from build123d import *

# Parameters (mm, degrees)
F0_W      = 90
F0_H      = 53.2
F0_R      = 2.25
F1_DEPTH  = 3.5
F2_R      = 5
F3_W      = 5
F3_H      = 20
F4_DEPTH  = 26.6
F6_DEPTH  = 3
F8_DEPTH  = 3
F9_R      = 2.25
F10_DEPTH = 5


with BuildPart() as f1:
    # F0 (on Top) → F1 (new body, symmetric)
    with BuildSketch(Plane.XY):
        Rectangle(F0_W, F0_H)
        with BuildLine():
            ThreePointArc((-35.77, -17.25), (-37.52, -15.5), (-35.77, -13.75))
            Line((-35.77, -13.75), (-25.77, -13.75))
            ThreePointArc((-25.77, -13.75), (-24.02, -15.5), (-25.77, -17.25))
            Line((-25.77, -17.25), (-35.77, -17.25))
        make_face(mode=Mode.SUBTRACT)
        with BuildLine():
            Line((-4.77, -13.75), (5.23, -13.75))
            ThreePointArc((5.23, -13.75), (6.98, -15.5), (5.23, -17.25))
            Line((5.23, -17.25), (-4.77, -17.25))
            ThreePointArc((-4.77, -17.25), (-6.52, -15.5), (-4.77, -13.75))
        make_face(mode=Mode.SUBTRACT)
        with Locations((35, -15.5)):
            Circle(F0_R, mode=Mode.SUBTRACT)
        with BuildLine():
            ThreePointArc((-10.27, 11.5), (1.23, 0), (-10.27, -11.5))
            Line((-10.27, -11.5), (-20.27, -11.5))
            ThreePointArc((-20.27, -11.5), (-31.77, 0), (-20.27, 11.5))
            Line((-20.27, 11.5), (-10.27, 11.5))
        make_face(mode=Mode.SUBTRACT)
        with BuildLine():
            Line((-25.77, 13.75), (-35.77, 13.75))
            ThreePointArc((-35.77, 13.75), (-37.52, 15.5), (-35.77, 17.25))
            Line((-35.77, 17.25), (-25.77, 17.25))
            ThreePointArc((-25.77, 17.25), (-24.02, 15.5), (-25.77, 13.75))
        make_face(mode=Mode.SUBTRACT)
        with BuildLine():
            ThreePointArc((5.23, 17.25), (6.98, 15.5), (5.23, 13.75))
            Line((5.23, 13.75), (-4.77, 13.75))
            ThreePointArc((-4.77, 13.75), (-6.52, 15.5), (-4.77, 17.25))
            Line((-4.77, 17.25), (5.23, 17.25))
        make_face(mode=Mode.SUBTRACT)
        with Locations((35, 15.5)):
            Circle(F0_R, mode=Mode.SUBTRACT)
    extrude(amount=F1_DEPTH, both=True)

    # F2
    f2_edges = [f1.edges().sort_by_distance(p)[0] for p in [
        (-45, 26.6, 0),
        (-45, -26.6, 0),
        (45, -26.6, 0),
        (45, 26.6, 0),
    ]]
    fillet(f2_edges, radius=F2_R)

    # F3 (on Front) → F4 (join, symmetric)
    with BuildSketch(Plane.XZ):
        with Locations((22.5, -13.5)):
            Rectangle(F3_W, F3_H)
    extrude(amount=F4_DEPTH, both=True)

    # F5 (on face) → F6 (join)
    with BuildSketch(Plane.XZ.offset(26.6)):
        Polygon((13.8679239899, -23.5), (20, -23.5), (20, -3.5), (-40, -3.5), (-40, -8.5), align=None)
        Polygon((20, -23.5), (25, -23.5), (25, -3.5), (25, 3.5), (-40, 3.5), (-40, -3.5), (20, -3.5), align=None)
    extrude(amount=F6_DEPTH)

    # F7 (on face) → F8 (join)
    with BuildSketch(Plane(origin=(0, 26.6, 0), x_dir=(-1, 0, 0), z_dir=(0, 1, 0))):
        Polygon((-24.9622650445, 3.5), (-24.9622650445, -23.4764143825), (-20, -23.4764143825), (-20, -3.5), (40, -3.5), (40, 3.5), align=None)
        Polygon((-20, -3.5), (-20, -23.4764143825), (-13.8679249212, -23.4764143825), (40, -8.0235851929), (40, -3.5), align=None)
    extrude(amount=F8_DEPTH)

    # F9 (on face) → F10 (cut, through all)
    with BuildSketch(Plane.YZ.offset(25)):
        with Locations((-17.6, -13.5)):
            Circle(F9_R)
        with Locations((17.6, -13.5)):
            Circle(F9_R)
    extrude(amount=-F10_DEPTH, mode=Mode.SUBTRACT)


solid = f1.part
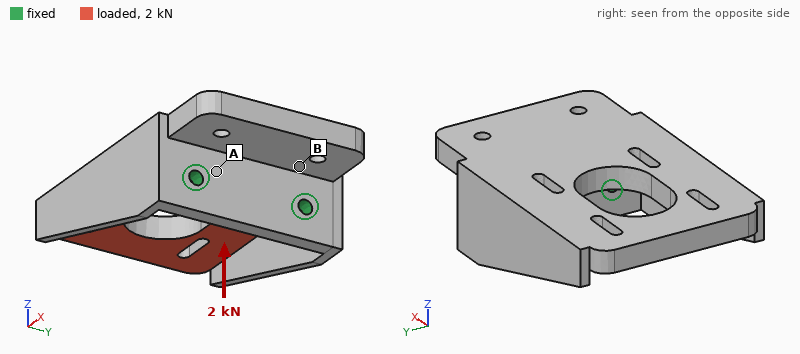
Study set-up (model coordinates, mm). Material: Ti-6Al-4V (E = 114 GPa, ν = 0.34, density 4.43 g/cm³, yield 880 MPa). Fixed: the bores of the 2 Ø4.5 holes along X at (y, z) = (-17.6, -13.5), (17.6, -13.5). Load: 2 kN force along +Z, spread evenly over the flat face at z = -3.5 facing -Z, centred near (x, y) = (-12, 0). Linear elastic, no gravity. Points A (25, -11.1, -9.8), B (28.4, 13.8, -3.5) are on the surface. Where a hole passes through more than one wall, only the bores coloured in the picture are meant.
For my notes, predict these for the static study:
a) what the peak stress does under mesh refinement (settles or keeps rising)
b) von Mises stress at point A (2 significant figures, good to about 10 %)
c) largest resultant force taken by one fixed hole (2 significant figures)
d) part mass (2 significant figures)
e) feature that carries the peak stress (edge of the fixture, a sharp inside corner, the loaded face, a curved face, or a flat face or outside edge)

keeps rising
110 MPa
1.0 kN
180 g
edge of the fixture
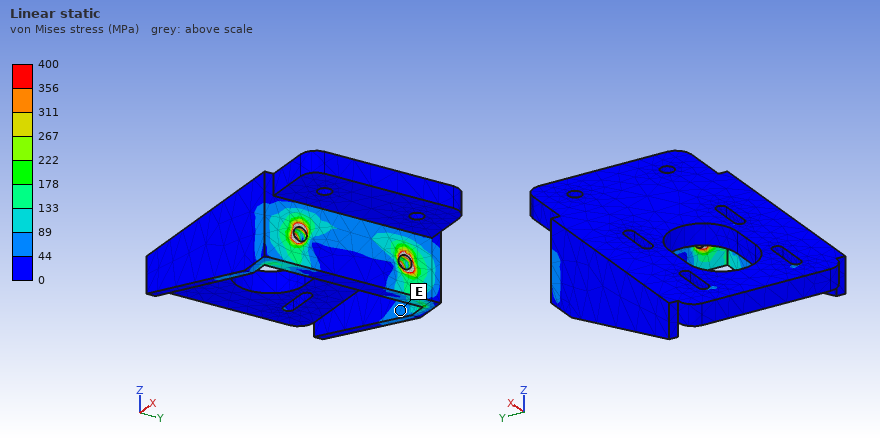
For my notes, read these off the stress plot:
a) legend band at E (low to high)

44 to 89 MPa
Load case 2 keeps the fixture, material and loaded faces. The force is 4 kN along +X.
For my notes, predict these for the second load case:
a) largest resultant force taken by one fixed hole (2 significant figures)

2.0 kN
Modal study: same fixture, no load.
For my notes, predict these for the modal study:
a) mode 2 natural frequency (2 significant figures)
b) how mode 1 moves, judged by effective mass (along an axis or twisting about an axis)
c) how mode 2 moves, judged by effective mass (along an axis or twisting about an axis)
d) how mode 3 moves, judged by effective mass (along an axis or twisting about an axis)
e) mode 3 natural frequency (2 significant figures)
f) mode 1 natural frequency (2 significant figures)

2200 Hz
along Z
along Y
along Y
4200 Hz
1200 Hz
